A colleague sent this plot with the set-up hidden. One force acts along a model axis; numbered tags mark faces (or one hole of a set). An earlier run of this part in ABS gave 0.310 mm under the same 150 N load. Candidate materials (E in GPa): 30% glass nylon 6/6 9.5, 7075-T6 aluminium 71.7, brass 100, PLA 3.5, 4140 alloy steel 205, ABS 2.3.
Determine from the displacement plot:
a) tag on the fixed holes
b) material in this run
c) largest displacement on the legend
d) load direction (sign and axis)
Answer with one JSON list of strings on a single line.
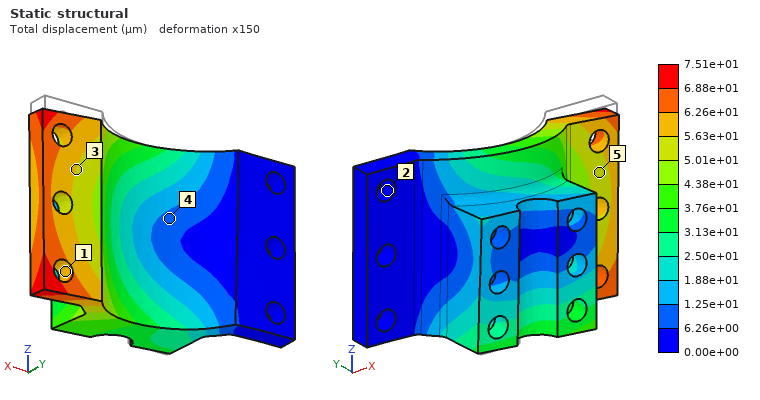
["2", "30% glass nylon 6/6", "7.51e+01 µm", "-Z"]
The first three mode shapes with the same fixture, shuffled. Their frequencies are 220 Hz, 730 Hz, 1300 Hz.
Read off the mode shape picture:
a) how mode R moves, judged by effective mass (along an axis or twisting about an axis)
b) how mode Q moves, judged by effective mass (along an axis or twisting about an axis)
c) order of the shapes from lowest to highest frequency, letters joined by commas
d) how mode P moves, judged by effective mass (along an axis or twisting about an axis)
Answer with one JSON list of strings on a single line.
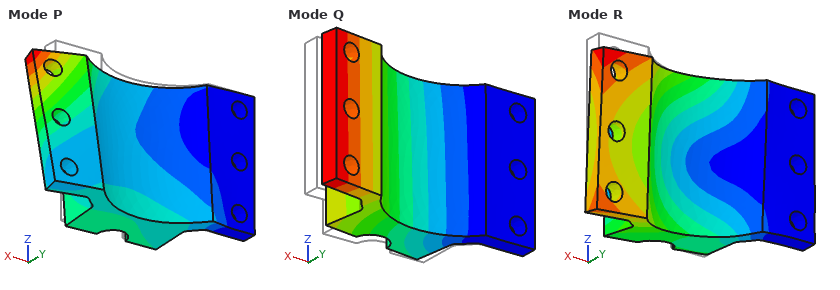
["along Z", "along Y", "Q, R, P", "along Z"]
